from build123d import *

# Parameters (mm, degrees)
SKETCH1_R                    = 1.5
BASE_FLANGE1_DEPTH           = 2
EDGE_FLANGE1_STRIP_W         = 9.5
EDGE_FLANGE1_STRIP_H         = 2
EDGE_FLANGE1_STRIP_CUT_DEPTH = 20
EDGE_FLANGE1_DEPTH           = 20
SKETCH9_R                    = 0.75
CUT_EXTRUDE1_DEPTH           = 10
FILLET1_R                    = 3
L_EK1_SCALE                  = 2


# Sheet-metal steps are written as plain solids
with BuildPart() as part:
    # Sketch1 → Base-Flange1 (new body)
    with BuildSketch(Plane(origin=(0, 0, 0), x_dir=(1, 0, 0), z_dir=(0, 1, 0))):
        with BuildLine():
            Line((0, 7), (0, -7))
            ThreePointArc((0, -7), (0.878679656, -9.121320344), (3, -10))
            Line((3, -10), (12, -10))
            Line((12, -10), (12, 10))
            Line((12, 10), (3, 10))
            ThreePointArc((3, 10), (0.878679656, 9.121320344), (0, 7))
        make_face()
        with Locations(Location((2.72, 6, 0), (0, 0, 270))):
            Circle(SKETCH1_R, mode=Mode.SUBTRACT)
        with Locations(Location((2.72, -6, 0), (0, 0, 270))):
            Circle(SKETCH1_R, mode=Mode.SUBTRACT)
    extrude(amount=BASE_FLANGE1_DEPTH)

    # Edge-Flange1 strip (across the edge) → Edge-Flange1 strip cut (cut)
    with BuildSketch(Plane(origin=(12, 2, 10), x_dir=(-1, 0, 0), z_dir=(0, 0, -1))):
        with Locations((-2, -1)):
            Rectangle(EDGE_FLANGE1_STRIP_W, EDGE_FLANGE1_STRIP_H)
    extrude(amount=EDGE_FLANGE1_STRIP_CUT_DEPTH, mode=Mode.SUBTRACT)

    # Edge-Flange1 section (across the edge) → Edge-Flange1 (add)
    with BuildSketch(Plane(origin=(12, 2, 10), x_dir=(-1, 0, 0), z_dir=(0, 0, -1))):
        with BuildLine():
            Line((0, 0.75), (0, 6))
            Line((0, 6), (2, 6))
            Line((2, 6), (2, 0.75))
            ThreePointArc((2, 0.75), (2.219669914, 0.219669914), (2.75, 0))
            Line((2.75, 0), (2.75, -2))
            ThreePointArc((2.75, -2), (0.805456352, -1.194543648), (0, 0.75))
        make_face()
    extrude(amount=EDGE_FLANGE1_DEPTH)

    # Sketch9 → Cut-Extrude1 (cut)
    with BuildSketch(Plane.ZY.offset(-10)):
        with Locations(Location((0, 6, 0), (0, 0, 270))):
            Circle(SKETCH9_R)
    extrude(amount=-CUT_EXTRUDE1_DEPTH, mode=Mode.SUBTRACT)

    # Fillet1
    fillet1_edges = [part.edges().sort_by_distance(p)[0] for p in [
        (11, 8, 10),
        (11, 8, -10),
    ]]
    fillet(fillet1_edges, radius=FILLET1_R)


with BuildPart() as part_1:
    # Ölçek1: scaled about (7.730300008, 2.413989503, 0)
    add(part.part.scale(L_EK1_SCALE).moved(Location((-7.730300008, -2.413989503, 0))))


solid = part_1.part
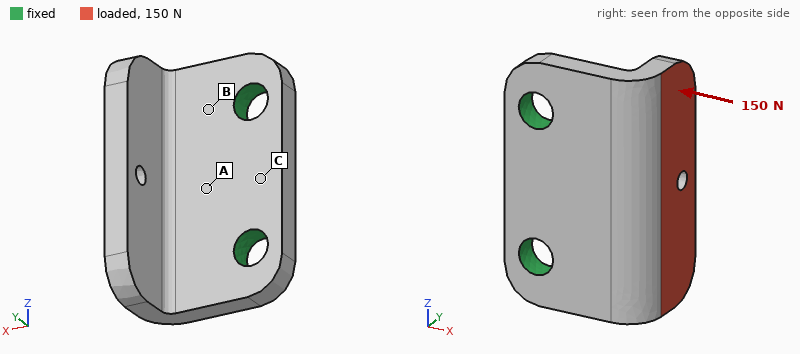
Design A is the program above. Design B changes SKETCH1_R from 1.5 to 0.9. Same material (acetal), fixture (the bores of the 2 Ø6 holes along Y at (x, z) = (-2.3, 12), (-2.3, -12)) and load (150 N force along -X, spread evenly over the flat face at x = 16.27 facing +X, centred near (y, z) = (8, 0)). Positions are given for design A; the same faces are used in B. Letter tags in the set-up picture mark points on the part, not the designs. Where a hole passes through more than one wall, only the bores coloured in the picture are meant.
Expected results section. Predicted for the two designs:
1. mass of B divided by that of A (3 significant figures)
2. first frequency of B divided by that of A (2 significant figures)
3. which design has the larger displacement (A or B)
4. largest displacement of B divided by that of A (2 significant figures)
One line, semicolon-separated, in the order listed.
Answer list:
1.03; 0.87; B; 1.2
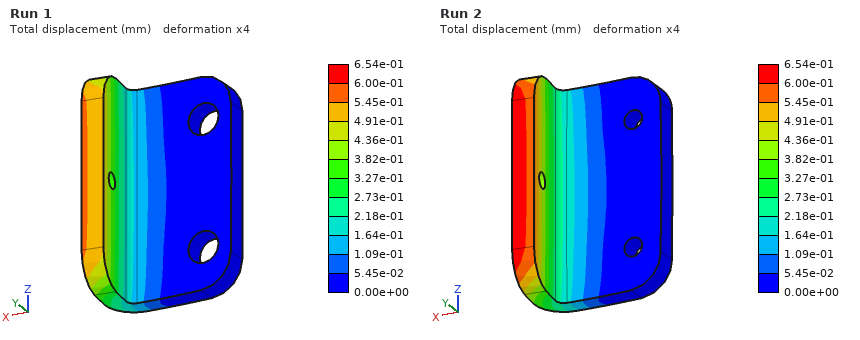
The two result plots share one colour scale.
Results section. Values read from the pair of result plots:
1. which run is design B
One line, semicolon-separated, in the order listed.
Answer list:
Run 2
